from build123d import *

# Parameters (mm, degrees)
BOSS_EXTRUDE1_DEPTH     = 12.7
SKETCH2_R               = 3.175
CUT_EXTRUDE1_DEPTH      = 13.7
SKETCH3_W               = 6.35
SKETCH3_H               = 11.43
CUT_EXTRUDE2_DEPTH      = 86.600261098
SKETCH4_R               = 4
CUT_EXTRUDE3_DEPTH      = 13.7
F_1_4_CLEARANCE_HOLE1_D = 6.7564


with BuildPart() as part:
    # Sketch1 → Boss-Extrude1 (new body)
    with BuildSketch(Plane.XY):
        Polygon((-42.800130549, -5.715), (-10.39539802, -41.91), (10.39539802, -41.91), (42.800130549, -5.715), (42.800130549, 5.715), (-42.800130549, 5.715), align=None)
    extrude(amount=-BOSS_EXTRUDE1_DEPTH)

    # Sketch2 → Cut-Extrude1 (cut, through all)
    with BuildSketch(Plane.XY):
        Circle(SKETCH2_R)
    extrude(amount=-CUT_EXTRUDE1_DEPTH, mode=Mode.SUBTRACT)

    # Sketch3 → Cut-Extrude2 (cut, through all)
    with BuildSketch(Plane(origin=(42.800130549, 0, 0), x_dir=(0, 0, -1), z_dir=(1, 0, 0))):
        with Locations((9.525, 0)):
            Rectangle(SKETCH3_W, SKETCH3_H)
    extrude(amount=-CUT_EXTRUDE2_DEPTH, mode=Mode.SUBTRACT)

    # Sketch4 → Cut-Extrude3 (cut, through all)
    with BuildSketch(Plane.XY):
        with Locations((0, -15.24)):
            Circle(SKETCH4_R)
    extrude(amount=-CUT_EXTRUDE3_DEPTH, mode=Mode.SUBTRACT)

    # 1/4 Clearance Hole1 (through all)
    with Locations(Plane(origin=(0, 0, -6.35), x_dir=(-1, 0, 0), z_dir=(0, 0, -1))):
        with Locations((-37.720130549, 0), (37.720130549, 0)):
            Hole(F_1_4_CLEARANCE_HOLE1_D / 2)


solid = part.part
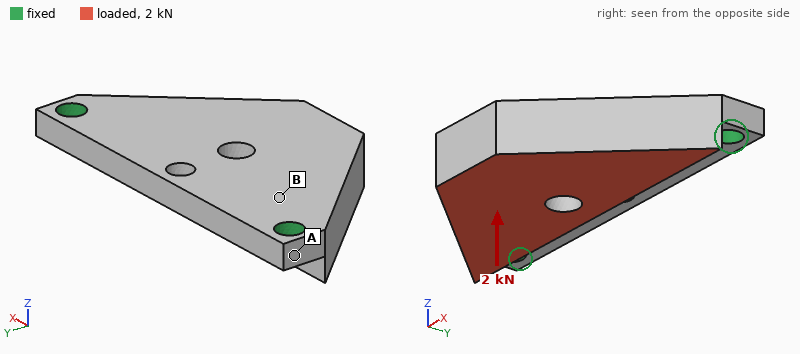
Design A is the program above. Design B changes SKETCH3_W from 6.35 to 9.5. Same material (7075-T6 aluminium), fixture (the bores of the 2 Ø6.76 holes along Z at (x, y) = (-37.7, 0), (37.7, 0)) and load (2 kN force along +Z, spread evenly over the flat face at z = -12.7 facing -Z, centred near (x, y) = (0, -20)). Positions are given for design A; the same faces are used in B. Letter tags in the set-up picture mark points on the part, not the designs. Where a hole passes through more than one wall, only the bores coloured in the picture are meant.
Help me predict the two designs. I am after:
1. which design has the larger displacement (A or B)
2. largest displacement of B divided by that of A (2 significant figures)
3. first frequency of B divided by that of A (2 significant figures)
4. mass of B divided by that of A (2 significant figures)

B
1.8
0.75
0.95
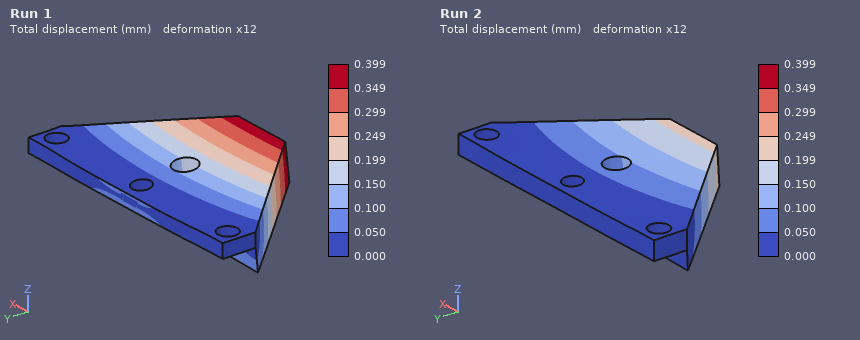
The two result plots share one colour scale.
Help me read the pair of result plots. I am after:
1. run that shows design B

Run 1
